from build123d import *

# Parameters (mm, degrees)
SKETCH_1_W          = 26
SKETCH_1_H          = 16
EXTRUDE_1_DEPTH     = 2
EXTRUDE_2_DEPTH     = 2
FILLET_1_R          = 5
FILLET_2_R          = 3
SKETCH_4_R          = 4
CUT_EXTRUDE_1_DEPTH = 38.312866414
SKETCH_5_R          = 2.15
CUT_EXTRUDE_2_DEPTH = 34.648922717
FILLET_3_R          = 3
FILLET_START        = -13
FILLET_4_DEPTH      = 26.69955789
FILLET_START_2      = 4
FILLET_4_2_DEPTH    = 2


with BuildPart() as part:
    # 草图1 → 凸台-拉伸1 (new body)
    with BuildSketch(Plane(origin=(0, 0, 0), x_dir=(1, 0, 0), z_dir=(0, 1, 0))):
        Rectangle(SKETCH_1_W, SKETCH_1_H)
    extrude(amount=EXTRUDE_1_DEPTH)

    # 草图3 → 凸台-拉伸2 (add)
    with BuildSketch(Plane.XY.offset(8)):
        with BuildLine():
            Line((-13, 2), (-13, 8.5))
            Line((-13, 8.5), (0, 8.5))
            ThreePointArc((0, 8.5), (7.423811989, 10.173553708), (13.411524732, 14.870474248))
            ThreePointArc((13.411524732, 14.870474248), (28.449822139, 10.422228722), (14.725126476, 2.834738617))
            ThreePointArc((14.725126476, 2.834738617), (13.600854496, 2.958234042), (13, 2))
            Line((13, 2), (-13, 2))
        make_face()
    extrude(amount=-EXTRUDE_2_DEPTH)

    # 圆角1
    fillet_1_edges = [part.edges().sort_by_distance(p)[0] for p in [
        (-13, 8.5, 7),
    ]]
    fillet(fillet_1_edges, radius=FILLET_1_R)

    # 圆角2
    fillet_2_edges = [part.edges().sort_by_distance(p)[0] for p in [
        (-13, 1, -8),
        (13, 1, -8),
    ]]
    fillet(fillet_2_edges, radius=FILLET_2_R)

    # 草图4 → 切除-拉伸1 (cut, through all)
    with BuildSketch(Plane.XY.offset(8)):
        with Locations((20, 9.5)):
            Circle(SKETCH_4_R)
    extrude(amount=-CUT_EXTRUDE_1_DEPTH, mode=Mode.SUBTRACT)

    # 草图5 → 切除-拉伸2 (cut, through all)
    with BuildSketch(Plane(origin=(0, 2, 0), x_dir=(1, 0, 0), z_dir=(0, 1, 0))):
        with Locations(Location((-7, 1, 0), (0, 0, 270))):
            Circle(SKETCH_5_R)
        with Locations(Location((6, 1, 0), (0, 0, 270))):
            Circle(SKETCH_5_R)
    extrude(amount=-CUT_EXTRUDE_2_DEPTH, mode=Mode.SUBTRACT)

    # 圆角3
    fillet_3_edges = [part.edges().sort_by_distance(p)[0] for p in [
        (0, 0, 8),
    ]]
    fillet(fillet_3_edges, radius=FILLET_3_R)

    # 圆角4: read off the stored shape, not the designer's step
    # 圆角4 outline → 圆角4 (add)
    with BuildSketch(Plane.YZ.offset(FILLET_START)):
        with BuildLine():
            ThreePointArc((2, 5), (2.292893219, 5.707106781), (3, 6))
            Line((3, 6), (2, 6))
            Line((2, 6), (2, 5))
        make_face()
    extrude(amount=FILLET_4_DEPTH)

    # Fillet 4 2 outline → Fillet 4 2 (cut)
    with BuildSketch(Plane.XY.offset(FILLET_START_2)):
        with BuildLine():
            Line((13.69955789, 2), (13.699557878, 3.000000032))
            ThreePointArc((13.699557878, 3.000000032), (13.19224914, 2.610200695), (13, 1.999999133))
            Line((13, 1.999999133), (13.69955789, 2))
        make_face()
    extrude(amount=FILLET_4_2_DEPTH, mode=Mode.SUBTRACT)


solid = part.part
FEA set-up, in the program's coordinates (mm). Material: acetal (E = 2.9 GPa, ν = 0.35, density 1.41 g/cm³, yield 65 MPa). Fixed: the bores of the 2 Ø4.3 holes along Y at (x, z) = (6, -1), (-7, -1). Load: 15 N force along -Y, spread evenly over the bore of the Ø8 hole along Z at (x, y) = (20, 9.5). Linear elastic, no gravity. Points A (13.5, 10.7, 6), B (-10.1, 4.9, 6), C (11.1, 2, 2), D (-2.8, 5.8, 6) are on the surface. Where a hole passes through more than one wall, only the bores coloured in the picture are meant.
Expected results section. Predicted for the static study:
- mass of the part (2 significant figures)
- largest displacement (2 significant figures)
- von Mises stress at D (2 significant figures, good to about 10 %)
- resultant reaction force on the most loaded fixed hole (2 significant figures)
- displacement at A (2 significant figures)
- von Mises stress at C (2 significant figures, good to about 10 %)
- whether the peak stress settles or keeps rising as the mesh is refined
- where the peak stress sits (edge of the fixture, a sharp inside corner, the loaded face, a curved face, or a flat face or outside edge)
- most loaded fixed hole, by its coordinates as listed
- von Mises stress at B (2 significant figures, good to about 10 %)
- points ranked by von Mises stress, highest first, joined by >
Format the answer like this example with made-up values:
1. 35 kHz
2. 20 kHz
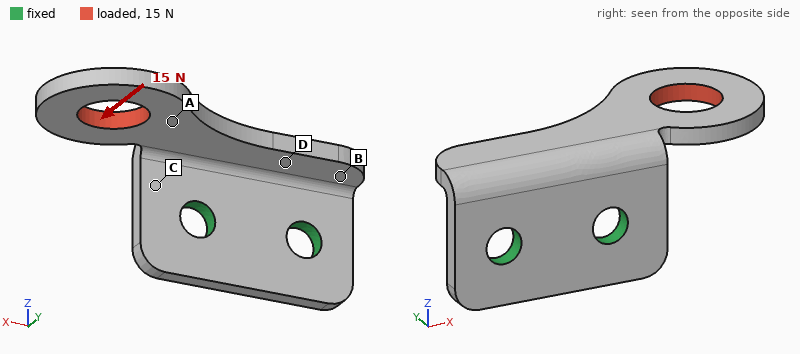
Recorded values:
1. 2.0 g
2. 0.49 mm
3. 5.1 MPa
4. 26 N
5. 0.24 mm
6. 9.4 MPa
7. keeps rising
8. edge of the fixture
9. (6, -1)
10. 3.1 MPa
11. C > D > B > A
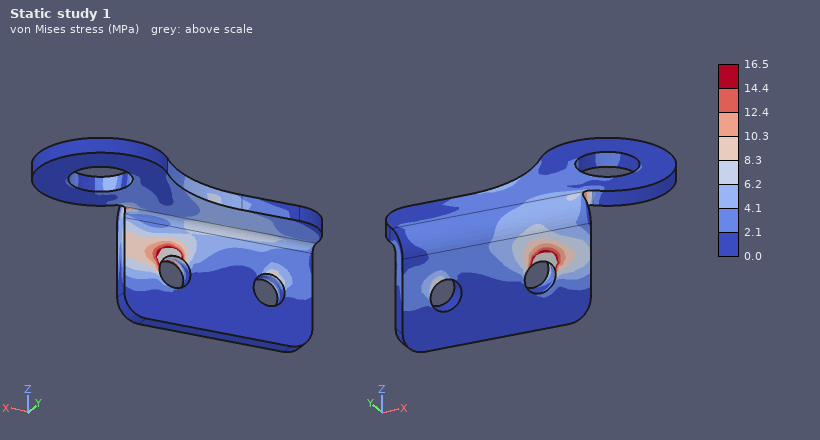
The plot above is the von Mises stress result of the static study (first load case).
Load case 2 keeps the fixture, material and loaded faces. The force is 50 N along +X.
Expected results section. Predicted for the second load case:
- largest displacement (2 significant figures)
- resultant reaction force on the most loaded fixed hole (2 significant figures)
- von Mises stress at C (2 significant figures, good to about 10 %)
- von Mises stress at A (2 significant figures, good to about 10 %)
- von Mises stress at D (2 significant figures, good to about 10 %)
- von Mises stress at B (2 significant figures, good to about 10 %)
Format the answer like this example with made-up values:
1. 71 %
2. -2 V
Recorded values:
1. 0.52 mm
2. 43 N
3. 8.6 MPa
4. 3.1 MPa
5. 7.8 MPa
6. 4.5 MPa
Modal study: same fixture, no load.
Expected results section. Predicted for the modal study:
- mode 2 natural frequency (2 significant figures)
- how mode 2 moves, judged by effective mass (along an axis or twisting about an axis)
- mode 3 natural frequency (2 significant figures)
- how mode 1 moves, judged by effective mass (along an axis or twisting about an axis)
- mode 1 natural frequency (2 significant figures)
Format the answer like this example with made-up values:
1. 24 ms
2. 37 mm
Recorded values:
1. 1600 Hz
2. along Y
3. 2000 Hz
4. along Z
5. 770 Hz
